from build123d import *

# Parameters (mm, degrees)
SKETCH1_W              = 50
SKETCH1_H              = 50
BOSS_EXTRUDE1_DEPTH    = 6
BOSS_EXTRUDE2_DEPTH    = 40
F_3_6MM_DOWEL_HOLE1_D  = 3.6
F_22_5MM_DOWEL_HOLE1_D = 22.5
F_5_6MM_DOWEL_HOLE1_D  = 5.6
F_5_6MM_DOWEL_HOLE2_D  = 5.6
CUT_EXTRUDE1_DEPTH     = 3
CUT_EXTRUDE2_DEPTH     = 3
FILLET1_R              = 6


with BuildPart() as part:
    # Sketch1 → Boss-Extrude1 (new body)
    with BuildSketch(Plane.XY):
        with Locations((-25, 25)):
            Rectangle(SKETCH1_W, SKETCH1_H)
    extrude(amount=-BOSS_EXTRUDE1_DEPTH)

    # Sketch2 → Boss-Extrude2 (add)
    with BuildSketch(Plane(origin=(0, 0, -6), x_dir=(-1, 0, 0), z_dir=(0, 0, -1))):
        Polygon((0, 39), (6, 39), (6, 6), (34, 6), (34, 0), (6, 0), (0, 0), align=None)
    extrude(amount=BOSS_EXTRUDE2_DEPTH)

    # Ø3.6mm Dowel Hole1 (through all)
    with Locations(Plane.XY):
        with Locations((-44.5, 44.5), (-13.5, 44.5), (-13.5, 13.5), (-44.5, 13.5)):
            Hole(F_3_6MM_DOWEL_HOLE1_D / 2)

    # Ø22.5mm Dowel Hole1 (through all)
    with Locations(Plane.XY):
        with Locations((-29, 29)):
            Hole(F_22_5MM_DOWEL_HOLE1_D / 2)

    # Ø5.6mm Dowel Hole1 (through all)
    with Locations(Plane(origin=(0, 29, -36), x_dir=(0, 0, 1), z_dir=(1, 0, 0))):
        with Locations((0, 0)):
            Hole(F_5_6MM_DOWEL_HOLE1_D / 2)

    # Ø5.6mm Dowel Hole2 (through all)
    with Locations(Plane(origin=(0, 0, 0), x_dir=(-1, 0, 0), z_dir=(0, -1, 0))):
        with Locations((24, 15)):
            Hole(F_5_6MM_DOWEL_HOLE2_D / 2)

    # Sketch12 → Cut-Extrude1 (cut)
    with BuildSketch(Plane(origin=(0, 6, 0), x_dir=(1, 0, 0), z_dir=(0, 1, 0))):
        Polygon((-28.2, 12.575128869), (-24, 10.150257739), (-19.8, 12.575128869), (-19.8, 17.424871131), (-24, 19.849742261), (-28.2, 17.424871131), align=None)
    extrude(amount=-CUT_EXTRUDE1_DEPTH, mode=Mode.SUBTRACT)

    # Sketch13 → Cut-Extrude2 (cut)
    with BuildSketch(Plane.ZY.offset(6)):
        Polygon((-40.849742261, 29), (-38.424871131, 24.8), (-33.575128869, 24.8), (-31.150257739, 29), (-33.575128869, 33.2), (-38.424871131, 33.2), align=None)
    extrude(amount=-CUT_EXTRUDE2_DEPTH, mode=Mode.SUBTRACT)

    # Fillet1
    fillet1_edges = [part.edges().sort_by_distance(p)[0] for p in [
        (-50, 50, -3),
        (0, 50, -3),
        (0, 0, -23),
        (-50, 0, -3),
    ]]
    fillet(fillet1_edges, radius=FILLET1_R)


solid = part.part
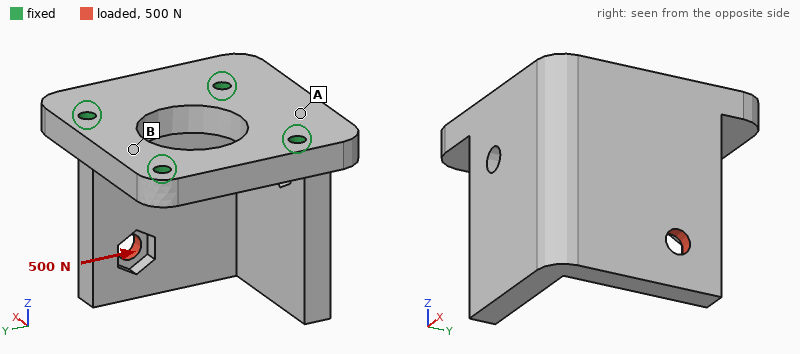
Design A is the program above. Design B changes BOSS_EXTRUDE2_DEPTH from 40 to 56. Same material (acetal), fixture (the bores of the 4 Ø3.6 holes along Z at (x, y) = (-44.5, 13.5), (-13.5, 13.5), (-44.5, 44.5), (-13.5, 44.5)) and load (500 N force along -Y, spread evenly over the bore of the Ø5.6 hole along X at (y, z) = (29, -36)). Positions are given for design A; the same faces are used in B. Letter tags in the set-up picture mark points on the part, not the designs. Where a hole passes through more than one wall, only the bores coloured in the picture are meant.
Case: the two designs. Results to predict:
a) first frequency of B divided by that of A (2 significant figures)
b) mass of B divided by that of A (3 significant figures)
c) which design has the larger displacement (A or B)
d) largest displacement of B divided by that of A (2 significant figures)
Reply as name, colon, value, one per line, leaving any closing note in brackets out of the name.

first frequency of B divided by that of A: 0.64
mass of B divided by that of A: 1.23
which design has the larger displacement: B
largest displacement of B divided by that of A: 1.3
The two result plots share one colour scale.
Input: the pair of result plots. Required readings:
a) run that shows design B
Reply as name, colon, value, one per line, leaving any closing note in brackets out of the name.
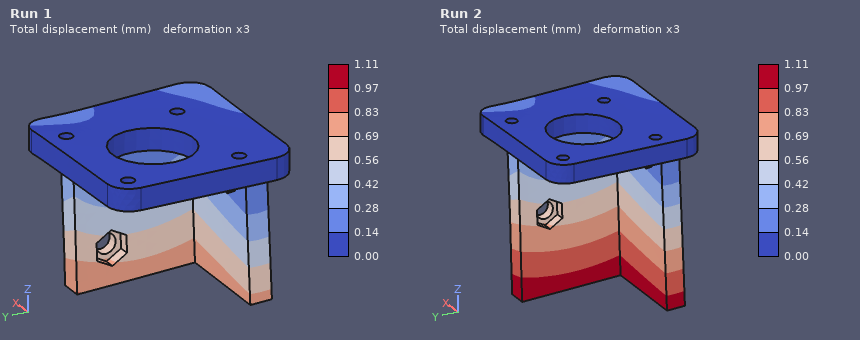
run that shows design B: Run 2
